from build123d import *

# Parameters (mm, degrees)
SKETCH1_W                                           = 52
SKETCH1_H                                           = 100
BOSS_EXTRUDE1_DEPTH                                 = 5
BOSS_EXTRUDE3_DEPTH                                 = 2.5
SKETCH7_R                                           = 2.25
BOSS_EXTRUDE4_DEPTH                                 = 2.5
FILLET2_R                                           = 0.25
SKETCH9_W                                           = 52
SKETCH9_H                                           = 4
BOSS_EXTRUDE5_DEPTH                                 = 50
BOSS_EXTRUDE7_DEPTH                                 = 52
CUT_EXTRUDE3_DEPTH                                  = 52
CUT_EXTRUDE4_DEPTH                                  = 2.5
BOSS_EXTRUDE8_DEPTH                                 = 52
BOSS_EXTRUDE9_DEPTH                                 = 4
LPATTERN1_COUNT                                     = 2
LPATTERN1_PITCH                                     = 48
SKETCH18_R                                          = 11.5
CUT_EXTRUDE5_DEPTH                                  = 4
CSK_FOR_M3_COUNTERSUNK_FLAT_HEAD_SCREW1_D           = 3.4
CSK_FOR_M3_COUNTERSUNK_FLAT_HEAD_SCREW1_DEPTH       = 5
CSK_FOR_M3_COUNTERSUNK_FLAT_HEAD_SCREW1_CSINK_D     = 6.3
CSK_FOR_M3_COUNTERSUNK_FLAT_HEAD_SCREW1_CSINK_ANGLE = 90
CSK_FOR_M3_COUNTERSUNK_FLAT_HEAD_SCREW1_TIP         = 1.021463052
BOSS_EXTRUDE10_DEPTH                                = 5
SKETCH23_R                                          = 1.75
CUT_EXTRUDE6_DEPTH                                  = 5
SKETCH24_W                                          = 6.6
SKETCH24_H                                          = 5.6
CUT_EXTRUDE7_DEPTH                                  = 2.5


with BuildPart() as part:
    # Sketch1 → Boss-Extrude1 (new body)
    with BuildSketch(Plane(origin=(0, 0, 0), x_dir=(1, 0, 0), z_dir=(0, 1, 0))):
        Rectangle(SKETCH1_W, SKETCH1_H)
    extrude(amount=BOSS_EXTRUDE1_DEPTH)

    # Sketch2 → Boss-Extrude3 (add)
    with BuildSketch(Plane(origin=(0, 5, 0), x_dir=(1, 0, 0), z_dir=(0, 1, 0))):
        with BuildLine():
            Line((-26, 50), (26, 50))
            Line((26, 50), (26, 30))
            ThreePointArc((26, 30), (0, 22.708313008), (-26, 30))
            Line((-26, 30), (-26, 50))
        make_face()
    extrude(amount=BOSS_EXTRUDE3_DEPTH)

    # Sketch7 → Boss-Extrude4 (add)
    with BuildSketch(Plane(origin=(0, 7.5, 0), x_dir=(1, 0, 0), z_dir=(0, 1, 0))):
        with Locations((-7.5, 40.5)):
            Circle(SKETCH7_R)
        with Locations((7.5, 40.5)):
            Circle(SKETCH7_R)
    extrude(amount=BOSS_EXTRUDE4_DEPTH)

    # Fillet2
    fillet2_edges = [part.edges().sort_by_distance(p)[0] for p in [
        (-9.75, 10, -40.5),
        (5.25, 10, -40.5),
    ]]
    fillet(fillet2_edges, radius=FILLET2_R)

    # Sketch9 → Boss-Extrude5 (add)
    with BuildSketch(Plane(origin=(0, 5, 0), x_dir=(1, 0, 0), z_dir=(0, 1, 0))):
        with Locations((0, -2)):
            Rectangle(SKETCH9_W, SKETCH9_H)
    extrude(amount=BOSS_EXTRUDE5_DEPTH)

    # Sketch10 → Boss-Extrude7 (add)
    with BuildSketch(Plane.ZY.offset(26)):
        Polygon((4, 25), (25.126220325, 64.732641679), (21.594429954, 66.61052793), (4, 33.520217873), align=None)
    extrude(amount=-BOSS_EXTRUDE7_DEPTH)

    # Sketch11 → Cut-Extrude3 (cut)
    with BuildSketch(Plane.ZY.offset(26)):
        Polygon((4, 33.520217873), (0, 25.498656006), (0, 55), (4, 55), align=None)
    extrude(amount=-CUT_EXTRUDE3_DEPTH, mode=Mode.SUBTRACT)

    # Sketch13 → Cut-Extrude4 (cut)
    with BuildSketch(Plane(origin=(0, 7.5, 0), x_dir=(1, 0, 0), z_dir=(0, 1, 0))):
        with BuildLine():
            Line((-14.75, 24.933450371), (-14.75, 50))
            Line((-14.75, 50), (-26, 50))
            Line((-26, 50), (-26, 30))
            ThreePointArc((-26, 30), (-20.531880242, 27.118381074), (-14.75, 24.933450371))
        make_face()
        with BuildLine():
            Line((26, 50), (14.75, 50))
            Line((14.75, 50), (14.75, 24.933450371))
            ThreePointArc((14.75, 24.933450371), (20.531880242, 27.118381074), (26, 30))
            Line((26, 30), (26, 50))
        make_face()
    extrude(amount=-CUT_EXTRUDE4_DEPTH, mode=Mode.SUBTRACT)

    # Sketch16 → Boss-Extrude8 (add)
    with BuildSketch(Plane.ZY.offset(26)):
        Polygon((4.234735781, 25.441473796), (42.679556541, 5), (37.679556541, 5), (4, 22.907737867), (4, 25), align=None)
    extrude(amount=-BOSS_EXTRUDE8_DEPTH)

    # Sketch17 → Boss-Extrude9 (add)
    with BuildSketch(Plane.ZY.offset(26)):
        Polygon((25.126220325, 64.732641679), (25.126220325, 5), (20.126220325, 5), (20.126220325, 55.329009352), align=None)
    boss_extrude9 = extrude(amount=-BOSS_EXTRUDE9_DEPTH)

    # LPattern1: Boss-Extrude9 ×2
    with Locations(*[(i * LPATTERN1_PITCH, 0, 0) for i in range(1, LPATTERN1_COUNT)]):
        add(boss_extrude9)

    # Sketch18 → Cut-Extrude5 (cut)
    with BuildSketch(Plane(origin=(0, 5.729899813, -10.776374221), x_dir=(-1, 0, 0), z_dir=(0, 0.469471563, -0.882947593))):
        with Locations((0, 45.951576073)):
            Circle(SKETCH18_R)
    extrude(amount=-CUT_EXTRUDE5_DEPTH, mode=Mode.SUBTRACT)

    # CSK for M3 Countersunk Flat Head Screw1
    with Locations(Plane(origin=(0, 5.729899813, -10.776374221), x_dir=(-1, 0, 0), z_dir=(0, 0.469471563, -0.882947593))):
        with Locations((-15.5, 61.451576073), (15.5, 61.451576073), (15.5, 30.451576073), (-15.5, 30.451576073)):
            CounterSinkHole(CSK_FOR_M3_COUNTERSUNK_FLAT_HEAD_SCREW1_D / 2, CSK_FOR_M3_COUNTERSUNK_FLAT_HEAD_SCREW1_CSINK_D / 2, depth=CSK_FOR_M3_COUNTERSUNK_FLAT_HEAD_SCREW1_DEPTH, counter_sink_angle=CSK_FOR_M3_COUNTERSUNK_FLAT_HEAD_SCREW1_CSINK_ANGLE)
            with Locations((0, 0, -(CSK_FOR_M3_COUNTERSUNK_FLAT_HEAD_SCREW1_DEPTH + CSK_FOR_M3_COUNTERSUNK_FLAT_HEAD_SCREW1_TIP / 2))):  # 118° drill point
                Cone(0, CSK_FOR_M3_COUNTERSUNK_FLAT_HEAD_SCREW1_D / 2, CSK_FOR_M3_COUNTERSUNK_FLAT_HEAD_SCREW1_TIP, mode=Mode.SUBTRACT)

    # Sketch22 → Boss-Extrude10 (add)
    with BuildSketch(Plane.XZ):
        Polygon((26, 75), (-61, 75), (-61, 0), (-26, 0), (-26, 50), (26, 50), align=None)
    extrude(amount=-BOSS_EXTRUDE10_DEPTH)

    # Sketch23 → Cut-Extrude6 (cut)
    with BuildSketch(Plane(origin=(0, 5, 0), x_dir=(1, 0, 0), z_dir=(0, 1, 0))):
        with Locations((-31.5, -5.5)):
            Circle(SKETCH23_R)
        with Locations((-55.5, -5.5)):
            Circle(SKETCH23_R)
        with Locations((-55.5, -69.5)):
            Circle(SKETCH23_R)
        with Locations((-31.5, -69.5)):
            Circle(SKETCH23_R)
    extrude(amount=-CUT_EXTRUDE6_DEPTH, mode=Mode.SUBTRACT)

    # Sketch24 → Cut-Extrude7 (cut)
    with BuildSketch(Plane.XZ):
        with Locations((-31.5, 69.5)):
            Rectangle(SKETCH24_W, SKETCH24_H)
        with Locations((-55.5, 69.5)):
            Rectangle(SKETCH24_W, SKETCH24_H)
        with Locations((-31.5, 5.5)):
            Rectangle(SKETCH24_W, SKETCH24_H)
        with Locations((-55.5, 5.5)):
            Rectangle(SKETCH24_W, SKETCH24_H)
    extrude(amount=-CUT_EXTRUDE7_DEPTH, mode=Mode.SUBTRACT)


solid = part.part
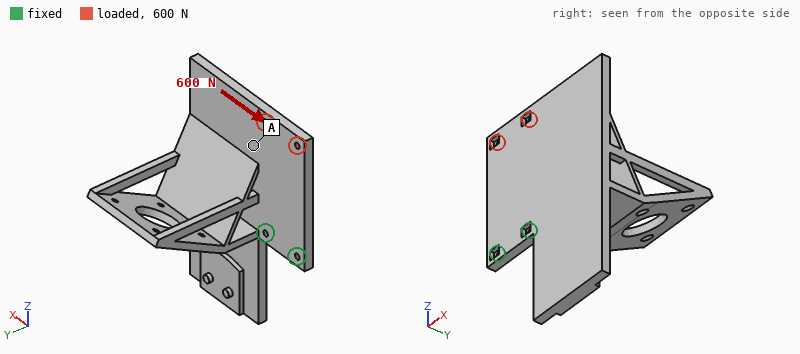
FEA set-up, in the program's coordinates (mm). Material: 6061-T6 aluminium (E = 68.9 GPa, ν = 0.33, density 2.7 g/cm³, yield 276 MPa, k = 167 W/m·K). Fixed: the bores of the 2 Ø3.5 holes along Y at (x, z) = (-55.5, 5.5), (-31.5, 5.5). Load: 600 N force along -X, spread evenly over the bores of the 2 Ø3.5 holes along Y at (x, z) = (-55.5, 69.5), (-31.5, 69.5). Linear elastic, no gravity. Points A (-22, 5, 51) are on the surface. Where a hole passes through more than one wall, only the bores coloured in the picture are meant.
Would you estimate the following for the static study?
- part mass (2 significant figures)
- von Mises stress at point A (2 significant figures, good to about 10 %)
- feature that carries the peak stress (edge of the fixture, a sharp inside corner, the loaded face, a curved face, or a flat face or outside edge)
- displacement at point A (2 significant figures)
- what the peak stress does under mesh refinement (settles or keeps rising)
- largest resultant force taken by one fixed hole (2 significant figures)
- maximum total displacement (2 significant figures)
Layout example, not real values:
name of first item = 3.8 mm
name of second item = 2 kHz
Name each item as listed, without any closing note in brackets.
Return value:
part mass = 180 g
von Mises stress at point A = 5.9 MPa
feature that carries the peak stress = edge of the fixture
displacement at point A = 0.049 mm
what the peak stress does under mesh refinement = keeps rising
largest resultant force taken by one fixed hole = 1.5 kN
maximum total displacement = 0.11 mm
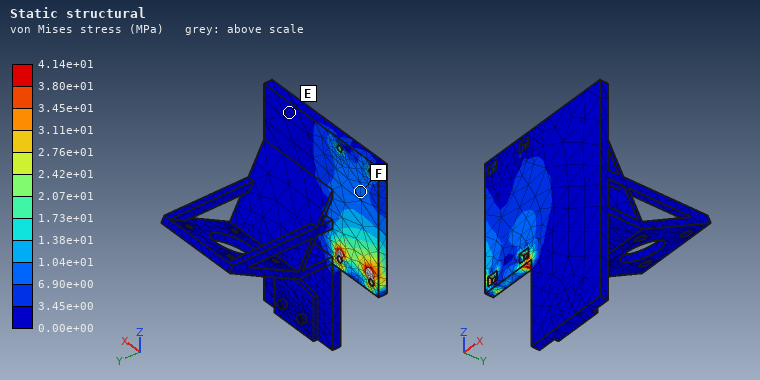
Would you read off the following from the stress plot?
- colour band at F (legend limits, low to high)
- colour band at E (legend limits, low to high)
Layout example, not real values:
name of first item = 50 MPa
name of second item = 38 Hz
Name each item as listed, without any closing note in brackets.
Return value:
colour band at F = 6.90e+00 to 1.04e+01 MPa
colour band at E = 0.00e+00 to 3.45e+00 MPa
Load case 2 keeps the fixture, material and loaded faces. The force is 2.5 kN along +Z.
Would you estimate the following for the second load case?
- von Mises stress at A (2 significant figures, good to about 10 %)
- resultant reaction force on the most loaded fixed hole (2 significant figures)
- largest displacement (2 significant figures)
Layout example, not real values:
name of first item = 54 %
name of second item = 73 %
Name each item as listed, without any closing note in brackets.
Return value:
von Mises stress at A = 16 MPa
resultant reaction force on the most loaded fixed hole = 1.3 kN
largest displacement = 0.14 mm
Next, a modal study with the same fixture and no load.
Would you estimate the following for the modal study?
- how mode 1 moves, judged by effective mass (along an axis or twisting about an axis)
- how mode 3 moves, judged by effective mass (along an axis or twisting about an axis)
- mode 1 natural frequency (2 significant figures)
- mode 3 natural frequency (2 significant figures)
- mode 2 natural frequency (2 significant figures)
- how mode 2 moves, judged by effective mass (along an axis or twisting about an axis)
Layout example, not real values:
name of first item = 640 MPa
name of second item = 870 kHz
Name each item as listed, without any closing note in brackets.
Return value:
how mode 1 moves, judged by effective mass = along Y
how mode 3 moves, judged by effective mass = along Y
mode 1 natural frequency = 370 Hz
mode 3 natural frequency = 1300 Hz
mode 2 natural frequency = 450 Hz
how mode 2 moves, judged by effective mass = along Y
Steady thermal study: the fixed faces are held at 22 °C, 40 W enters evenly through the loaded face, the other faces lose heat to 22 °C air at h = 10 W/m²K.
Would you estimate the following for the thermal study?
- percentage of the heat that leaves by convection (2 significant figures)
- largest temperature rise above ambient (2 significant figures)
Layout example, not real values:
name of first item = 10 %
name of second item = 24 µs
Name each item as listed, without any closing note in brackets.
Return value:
percentage of the heat that leaves by convection = 19 %
largest temperature rise above ambient = 73 K
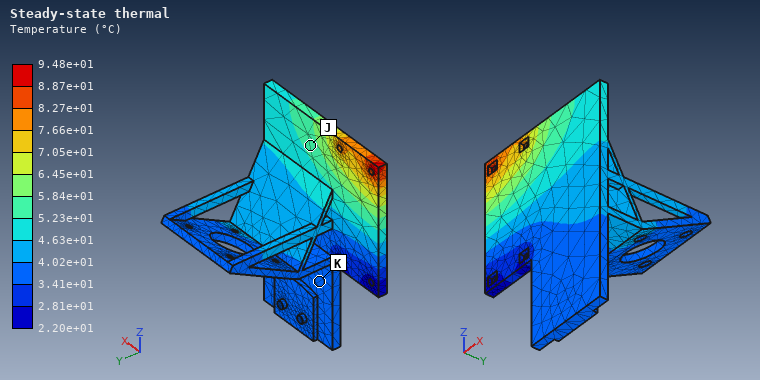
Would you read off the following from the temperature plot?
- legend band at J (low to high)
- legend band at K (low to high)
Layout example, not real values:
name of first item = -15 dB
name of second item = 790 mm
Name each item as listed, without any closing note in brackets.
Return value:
legend band at J = 5.23e+01 to 5.84e+01 °C
legend band at K = 3.41e+01 to 4.02e+01 °C
